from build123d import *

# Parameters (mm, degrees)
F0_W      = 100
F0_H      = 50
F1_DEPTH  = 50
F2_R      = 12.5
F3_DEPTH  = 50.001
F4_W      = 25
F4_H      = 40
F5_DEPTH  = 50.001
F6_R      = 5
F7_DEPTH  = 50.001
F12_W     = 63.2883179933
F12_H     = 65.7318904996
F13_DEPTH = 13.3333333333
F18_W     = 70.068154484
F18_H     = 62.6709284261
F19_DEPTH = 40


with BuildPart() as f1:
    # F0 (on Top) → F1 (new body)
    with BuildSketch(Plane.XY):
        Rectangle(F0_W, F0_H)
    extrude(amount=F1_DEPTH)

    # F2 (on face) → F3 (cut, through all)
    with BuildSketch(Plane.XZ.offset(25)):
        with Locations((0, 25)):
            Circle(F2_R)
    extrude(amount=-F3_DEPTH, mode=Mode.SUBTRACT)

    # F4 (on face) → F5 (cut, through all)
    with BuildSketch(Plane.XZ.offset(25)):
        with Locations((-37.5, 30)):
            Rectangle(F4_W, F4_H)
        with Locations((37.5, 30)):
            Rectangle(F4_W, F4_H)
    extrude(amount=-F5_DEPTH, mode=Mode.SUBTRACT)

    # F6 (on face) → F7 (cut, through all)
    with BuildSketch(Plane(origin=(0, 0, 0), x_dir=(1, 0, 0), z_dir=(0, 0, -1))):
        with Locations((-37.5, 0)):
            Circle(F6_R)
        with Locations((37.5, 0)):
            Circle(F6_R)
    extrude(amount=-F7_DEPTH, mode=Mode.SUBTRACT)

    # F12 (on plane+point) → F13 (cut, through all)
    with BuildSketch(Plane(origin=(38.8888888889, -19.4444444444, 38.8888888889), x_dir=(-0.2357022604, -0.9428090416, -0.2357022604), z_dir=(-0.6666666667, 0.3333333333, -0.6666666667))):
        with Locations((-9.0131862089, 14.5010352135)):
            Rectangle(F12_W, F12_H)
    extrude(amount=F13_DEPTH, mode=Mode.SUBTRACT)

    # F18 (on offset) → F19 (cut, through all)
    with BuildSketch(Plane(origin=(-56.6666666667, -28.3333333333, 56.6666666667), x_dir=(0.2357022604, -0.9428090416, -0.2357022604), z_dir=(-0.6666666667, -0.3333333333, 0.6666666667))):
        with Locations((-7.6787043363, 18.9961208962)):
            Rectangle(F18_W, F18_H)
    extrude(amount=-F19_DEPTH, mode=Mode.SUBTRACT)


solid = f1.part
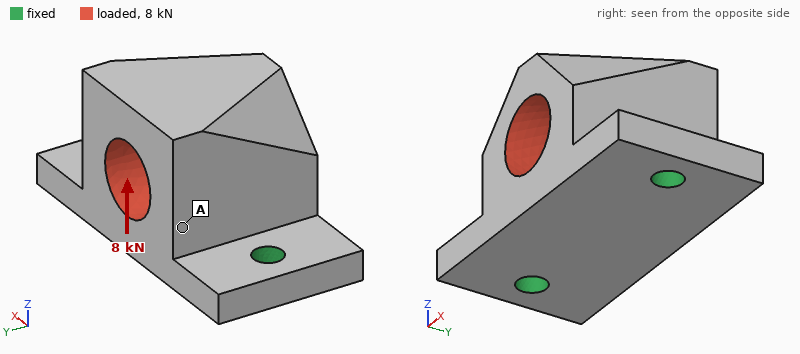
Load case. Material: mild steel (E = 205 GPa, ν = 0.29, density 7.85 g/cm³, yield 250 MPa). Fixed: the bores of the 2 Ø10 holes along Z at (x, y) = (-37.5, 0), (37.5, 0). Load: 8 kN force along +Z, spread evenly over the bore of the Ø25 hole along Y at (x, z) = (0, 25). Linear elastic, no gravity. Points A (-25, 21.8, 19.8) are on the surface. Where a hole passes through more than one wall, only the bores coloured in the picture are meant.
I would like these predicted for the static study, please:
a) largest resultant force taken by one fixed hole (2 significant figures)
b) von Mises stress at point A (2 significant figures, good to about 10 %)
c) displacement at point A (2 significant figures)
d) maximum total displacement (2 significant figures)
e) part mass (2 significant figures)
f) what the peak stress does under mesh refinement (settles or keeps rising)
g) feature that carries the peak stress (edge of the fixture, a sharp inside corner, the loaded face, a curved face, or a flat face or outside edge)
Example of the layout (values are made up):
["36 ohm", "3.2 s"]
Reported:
["4.3 kN", "9.1 MPa", "5.6 µm", "7.2 µm", "930 g", "keeps rising", "edge of the fixture"]
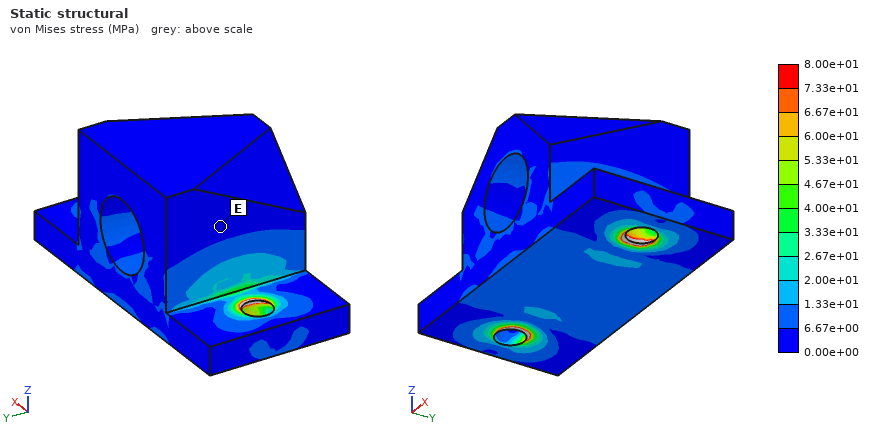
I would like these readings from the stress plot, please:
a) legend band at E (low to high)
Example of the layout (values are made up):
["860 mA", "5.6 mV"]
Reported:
["0.00e+00 to 6.67e+00 MPa"]
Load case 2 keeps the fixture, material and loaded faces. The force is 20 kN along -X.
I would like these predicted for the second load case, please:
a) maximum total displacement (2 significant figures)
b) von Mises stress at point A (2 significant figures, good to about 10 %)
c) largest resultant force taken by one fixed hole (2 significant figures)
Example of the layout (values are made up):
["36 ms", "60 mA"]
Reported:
["21 µm", "13 MPa", "12 kN"]
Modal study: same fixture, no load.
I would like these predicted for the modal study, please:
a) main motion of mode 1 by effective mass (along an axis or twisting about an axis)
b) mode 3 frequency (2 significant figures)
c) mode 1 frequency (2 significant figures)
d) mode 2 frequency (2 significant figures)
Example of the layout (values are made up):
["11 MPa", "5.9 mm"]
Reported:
["along Y", "6700 Hz", "2700 Hz", "6500 Hz"]
